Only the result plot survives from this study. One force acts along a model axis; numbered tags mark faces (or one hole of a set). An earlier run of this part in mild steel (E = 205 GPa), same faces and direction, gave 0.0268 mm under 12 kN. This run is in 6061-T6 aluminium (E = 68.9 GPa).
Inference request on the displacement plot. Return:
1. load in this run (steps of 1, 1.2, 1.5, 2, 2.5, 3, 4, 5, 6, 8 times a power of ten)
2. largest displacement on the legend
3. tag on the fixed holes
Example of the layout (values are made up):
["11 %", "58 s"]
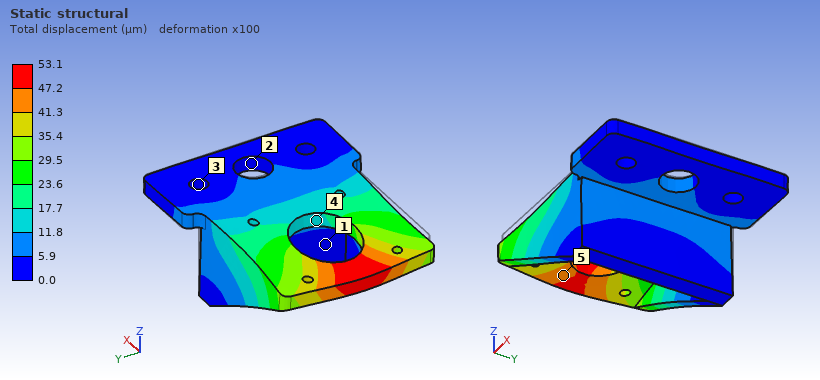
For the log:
["8 kN", "53.1 µm", "3"]
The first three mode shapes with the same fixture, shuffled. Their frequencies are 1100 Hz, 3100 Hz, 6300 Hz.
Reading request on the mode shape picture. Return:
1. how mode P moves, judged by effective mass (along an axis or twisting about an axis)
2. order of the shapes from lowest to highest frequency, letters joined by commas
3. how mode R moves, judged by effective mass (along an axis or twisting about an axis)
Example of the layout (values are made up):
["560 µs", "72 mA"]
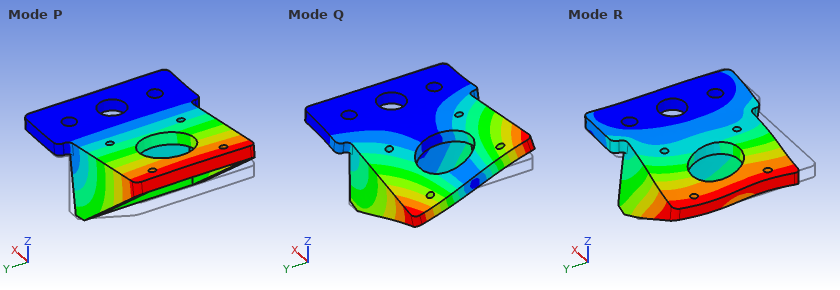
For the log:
["along Z", "P, Q, R", "along Y"]
